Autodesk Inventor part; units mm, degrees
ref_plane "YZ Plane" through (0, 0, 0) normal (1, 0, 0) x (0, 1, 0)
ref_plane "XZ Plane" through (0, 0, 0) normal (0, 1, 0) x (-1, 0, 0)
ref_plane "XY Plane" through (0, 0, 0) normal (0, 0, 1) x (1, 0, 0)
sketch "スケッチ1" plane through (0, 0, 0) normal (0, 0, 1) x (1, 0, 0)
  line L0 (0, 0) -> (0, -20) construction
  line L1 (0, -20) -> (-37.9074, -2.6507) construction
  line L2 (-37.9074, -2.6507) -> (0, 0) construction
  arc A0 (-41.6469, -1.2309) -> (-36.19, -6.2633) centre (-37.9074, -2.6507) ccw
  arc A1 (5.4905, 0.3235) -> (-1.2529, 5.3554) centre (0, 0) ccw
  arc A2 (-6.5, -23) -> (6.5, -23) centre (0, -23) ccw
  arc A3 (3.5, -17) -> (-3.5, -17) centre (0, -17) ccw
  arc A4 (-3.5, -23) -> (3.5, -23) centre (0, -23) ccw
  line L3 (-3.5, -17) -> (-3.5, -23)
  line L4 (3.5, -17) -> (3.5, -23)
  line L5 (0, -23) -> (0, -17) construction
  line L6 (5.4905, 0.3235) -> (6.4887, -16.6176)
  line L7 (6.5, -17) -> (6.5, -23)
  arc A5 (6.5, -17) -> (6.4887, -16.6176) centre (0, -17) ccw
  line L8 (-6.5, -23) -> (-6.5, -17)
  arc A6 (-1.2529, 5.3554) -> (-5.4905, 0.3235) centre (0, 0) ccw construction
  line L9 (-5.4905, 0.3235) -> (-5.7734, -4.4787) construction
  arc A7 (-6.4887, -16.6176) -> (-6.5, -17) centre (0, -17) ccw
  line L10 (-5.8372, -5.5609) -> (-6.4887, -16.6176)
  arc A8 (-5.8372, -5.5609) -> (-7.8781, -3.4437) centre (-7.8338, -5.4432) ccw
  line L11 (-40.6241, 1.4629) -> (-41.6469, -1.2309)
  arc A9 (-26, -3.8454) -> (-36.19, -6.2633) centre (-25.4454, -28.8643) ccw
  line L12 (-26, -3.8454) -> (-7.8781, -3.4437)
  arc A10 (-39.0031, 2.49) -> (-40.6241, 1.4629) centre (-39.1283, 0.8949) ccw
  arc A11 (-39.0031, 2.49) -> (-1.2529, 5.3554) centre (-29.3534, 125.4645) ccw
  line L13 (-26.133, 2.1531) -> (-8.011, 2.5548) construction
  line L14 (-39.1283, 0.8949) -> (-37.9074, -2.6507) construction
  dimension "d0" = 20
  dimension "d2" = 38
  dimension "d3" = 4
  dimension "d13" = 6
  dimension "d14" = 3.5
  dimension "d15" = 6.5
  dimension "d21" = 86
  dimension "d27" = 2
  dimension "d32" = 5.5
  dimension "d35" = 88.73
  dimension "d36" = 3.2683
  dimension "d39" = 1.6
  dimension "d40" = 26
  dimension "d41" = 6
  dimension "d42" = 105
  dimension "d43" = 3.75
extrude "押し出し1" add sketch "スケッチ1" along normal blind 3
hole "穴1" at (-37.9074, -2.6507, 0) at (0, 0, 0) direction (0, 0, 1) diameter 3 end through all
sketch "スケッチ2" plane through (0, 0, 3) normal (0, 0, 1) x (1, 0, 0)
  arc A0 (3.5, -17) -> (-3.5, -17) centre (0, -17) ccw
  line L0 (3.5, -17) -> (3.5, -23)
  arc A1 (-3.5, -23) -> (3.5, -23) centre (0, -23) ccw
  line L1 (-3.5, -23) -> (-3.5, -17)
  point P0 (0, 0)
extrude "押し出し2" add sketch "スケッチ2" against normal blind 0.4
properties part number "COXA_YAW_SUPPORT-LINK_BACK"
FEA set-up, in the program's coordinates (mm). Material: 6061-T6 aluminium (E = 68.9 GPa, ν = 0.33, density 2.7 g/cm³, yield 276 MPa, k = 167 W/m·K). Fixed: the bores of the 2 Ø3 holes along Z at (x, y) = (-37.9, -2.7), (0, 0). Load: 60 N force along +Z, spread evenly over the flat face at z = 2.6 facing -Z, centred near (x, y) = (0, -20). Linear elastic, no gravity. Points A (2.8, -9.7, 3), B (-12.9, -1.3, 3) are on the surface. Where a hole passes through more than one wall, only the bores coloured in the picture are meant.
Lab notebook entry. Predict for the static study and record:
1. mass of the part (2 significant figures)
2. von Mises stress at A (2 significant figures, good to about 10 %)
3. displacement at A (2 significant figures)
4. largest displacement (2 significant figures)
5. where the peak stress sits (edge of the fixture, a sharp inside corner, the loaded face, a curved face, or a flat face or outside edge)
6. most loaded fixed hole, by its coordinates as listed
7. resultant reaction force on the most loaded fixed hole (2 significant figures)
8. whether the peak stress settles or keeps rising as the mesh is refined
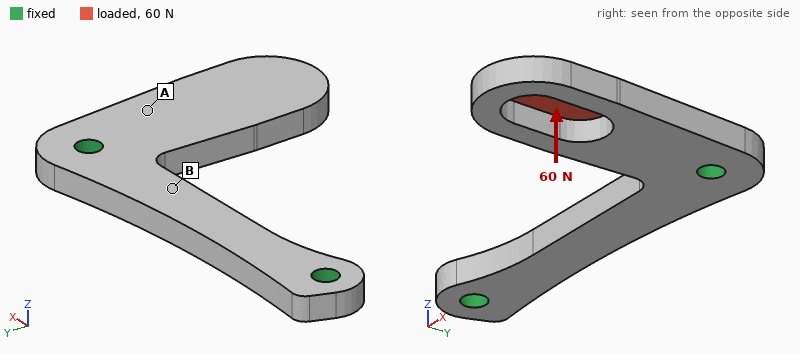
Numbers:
4.6 g
33 MPa
0.024 mm
0.15 mm
edge of the fixture
(0, 0)
62 N
keeps rising
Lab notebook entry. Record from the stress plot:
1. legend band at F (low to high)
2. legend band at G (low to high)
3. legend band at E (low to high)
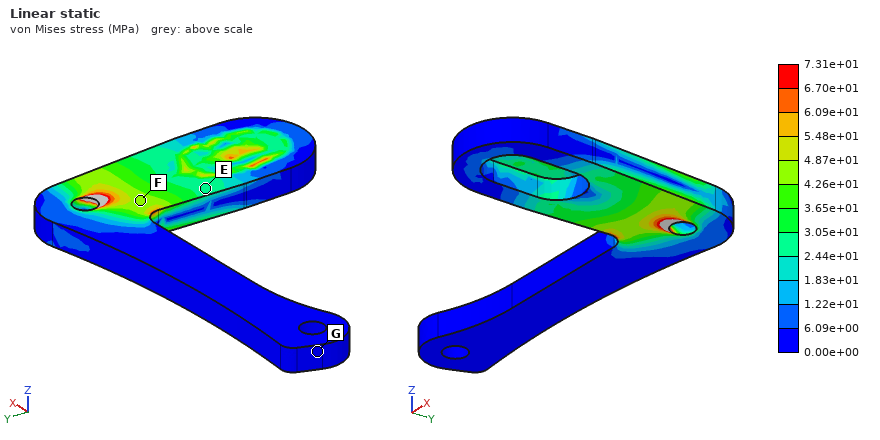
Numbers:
4.26e+01 to 4.87e+01 MPa
0.00e+00 to 6.09e+00 MPa
2.44e+01 to 3.05e+01 MPa
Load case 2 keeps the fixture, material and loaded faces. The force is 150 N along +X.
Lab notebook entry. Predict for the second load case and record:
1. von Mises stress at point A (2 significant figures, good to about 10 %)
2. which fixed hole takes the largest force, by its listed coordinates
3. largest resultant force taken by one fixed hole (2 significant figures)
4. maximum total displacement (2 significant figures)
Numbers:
17 MPa
(0, 0)
150 N
56 µm
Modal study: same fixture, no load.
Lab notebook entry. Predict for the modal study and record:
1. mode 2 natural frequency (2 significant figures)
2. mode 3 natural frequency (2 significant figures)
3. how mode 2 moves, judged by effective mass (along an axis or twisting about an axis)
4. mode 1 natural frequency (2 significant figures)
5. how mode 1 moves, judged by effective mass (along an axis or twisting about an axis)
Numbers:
8400 Hz
11 kHz
along X
3500 Hz
along Z
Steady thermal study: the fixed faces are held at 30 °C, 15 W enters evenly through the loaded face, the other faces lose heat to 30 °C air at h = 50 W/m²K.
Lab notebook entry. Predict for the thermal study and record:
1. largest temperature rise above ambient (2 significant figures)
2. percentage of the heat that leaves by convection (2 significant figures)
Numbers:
67 K
11 %
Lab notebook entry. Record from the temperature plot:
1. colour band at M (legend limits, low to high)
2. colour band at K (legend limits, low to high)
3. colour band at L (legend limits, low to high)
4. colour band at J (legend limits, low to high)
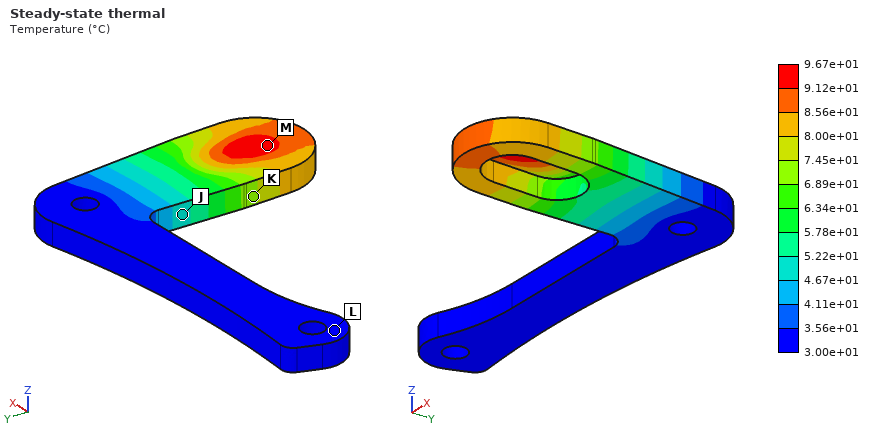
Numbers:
9.12e+01 to 9.67e+01 °C
6.89e+01 to 7.45e+01 °C
3.00e+01 to 3.56e+01 °C
4.67e+01 to 5.22e+01 °C
